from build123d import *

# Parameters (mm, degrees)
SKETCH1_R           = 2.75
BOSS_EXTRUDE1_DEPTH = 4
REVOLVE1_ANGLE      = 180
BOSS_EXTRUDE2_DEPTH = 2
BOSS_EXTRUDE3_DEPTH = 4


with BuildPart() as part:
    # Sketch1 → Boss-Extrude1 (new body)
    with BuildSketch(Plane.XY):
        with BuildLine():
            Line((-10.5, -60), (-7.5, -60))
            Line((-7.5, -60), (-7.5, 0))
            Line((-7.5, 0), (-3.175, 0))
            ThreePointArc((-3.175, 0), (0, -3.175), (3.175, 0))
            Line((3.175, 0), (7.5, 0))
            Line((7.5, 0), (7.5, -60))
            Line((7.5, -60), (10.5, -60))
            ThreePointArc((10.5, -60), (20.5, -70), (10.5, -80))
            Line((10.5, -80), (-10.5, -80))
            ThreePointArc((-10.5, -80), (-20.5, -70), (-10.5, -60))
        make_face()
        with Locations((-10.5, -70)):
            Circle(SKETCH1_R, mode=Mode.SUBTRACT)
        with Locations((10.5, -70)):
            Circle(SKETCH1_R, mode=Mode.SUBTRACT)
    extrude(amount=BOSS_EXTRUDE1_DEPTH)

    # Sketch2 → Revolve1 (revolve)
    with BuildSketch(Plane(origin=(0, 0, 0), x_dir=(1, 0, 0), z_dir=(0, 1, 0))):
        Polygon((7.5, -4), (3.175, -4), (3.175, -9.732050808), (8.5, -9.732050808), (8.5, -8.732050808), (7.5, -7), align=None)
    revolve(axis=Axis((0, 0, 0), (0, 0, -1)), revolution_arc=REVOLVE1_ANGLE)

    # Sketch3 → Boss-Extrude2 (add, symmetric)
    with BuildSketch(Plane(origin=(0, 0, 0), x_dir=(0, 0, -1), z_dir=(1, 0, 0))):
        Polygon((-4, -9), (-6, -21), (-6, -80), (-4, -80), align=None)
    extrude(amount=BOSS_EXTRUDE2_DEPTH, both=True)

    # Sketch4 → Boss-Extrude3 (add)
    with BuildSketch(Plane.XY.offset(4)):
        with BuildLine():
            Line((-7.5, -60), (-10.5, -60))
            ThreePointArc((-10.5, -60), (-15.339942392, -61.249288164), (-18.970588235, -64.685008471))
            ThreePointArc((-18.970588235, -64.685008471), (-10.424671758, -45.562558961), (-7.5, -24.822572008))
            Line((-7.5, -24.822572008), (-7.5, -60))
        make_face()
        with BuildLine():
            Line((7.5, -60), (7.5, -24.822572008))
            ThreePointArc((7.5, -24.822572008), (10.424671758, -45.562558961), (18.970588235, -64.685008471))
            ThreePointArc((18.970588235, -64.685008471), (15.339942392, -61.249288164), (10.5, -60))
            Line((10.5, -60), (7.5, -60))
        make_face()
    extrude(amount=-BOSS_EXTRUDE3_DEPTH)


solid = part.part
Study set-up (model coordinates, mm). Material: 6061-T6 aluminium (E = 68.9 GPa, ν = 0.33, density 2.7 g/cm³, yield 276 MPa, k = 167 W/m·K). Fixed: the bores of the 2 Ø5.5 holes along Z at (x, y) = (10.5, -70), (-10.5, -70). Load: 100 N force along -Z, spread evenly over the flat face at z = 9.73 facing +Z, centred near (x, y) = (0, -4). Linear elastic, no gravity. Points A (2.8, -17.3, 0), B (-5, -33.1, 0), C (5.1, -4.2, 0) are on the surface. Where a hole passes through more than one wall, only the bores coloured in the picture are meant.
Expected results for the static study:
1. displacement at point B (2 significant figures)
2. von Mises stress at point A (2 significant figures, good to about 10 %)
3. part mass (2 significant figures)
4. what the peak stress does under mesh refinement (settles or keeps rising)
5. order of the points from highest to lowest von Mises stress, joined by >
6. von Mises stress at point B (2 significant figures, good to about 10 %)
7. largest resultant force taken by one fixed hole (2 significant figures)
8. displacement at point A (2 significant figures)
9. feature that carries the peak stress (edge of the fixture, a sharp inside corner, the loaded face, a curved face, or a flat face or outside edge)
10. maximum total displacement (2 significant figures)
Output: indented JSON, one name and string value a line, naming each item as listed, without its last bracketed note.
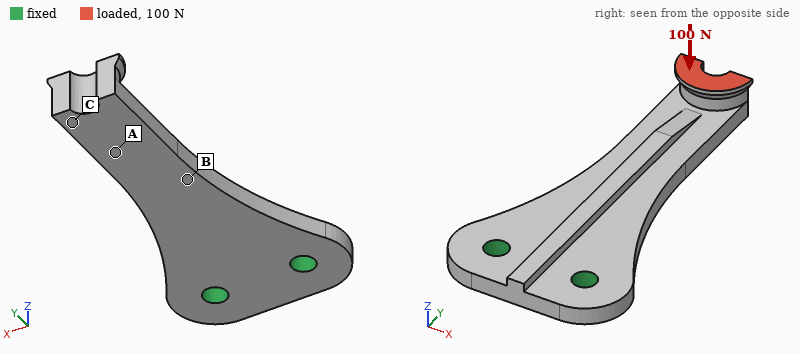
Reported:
{
  "displacement at point B": "0.24 mm",
  "von Mises stress at point A": "25 MPa",
  "part mass": "22 g",
  "what the peak stress does under mesh refinement": "keeps rising",
  "order of the points from highest to lowest von Mises stress, joined by >": "B > A > C",
  "von Mises stress at point B": "45 MPa",
  "largest resultant force taken by one fixed hole": "69 N",
  "displacement at point A": "0.47 mm",
  "feature that carries the peak stress": "edge of the fixture",
  "maximum total displacement": "0.77 mm"
}
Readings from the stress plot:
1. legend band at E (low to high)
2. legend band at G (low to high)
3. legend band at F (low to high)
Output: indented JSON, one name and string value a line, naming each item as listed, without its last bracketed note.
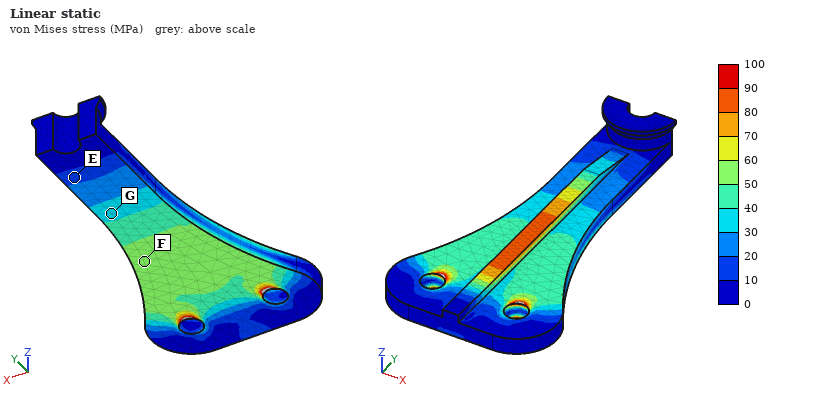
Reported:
{
  "legend band at E": "10 to 20 MPa",
  "legend band at G": "30 to 40 MPa",
  "legend band at F": "50 to 60 MPa"
}
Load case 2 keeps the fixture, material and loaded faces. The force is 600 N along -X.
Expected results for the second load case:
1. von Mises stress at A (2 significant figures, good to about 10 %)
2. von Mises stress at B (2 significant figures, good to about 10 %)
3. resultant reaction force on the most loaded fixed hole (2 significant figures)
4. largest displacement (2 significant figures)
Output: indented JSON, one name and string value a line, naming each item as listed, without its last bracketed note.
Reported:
{
  "von Mises stress at A": "78 MPa",
  "von Mises stress at B": "92 MPa",
  "resultant reaction force on the most loaded fixed hole": "1.7 kN",
  "largest displacement": "0.50 mm"
}
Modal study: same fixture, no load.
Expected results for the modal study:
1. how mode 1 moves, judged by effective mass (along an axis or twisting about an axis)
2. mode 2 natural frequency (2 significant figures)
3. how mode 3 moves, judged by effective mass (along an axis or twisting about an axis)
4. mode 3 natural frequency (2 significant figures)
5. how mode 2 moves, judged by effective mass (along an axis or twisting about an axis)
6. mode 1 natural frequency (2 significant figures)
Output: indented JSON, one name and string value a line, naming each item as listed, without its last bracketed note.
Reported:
{
  "how mode 1 moves, judged by effective mass": "along Z",
  "mode 2 natural frequency": "4000 Hz",
  "how mode 3 moves, judged by effective mass": "along Z",
  "mode 3 natural frequency": "4900 Hz",
  "how mode 2 moves, judged by effective mass": "along X",
  "mode 1 natural frequency": "920 Hz"
}
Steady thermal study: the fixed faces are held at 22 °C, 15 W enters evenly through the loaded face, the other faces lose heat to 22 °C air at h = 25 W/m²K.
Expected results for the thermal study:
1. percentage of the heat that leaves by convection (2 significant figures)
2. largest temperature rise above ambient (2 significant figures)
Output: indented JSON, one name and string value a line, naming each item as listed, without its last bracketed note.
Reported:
{
  "percentage of the heat that leaves by convection": "17 %",
  "largest temperature rise above ambient": "71 K"
}
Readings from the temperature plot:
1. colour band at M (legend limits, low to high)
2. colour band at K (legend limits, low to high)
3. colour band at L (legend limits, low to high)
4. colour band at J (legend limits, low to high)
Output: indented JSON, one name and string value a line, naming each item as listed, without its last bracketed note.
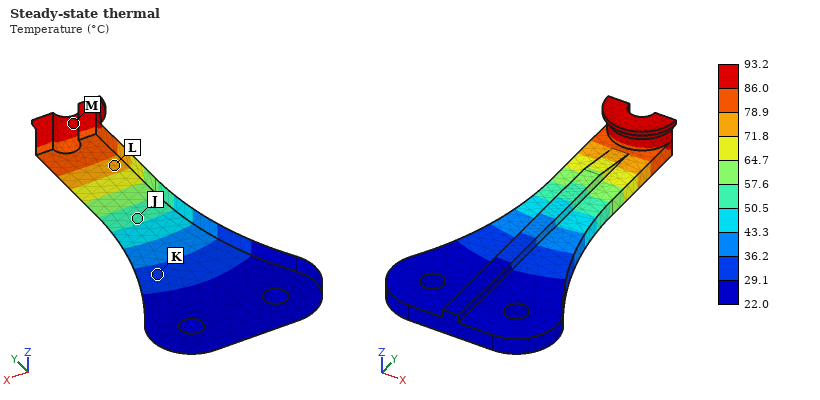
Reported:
{
  "colour band at M": "86.0 to 93.2 °C",
  "colour band at K": "29.1 to 36.2 °C",
  "colour band at L": "71.8 to 78.9 °C",
  "colour band at J": "50.5 to 57.6 °C"
}
